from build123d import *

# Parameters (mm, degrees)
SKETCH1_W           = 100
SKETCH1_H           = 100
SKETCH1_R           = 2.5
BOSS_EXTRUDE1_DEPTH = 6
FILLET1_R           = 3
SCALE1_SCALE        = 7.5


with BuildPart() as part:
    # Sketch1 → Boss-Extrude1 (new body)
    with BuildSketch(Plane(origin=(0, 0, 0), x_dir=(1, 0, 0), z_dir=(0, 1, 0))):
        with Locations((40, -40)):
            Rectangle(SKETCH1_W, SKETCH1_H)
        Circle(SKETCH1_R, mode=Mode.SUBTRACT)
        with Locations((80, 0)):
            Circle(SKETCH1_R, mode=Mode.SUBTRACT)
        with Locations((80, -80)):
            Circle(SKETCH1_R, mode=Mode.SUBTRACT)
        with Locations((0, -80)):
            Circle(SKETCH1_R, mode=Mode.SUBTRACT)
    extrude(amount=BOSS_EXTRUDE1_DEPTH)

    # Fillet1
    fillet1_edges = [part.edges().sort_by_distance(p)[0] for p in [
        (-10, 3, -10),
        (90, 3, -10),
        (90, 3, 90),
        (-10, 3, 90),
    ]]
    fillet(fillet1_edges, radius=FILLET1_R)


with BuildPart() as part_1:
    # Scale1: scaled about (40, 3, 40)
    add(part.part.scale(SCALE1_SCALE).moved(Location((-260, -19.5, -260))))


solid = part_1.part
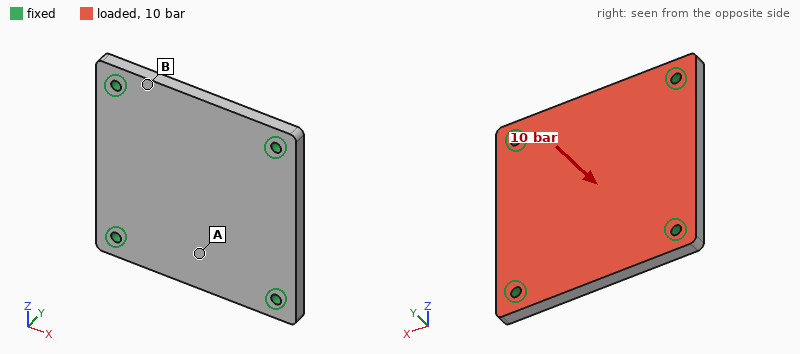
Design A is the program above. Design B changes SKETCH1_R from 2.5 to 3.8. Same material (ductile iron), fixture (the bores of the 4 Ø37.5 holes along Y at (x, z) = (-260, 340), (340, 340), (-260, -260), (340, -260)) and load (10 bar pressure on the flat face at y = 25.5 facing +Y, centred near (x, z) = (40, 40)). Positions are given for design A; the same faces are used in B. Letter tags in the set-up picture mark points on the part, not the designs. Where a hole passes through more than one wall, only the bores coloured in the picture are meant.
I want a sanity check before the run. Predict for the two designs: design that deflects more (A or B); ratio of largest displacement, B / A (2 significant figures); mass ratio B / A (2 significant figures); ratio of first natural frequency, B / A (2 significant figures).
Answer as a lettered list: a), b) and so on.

a) A
b) 0.85
c) 0.99
d) 1.1
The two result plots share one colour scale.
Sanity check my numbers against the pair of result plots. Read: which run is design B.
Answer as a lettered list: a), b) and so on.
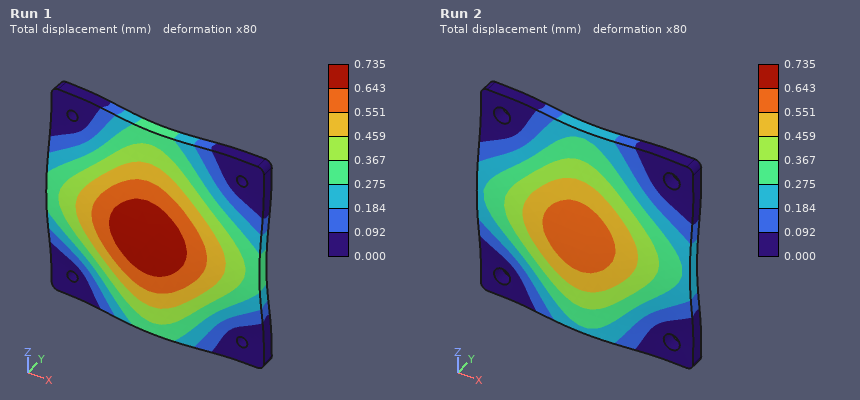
a) Run 2
